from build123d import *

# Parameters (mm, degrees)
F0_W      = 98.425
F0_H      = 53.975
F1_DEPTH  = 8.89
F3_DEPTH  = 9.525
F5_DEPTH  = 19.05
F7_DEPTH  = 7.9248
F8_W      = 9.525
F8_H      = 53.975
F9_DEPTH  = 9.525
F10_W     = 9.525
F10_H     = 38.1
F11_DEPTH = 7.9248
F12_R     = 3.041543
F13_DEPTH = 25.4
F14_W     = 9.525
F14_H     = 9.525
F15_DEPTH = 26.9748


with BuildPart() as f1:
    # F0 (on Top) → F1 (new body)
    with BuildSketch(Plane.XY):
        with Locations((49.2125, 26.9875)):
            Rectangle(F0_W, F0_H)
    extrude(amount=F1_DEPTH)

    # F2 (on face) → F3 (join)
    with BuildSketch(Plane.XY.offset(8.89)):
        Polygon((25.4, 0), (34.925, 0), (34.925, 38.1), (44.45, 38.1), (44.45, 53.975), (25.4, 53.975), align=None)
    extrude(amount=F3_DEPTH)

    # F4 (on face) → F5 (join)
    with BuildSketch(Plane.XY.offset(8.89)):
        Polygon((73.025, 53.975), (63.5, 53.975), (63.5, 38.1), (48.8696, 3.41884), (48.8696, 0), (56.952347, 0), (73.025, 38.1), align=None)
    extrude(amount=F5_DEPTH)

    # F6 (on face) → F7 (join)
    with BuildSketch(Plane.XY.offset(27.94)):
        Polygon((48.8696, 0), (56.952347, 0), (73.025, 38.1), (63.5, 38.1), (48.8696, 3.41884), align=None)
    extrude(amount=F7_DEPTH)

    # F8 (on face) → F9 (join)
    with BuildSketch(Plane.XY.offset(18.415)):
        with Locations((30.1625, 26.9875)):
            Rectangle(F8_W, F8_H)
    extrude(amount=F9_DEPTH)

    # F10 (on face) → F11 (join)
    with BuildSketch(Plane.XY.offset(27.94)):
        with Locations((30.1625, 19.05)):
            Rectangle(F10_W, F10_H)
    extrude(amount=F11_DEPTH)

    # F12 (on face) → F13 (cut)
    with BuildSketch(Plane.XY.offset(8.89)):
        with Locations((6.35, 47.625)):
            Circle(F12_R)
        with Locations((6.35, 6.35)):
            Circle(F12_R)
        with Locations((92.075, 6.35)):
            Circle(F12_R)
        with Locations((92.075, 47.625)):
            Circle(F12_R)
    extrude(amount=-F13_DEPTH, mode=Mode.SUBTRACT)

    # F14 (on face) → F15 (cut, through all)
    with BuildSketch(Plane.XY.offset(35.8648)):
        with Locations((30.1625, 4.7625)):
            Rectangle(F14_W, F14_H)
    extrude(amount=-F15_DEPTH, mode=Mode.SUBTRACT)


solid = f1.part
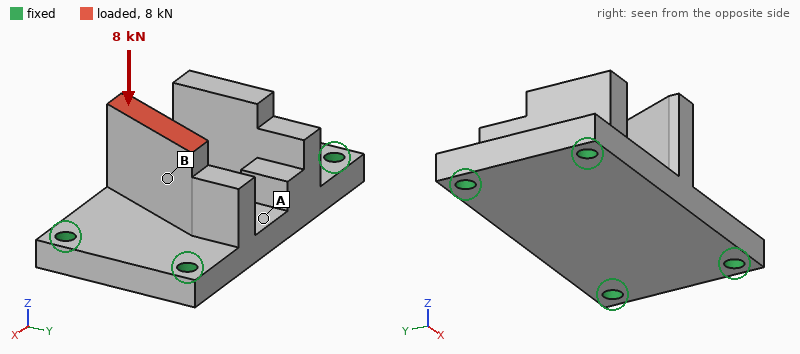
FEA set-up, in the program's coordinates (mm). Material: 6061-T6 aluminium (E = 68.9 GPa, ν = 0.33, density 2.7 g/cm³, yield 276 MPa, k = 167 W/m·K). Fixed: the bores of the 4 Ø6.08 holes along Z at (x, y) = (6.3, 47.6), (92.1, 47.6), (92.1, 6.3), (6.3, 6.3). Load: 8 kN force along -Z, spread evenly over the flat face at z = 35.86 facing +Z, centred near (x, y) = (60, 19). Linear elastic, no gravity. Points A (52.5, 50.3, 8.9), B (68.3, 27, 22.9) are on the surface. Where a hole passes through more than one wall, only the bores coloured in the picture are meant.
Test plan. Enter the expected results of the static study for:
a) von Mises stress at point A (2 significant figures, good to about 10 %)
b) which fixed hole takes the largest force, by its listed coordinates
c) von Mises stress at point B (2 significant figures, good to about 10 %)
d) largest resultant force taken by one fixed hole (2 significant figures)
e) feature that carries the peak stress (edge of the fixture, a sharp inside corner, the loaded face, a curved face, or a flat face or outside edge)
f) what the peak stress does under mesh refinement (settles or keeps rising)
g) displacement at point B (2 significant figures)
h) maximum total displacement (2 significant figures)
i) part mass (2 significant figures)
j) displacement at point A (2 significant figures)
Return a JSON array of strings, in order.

["58 MPa", "(92.1, 6.3)", "21 MPa", "3.4 kN", "edge of the fixture", "keeps rising", "0.10 mm", "0.20 mm", "190 g", "0.076 mm"]
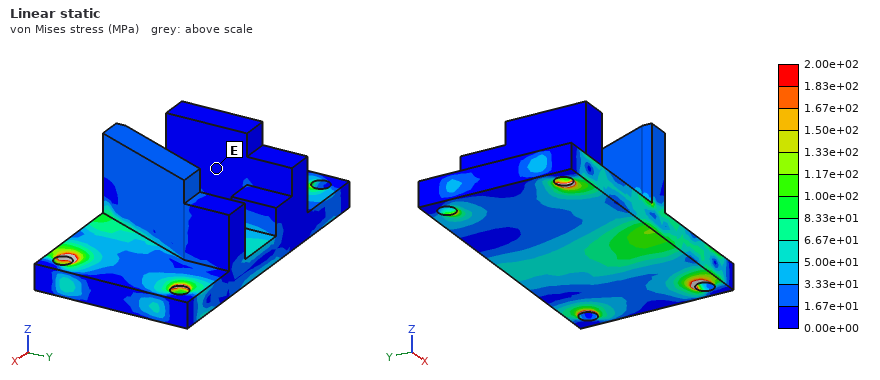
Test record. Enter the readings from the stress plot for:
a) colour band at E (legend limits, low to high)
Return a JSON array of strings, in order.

["0.00e+00 to 1.67e+01 MPa"]
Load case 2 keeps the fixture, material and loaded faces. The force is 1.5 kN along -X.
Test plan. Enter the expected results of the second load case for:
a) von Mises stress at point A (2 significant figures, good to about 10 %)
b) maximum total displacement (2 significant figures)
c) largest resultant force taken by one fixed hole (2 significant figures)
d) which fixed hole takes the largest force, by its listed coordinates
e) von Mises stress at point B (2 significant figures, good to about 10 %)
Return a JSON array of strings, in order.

["16 MPa", "0.10 mm", "640 N", "(92.1, 6.3)", "33 MPa"]
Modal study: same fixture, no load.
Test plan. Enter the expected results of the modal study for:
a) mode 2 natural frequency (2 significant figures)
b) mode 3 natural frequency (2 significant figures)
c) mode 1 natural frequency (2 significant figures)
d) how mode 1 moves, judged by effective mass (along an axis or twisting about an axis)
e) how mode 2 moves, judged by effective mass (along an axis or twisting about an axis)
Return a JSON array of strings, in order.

["5400 Hz", "7400 Hz", "3900 Hz", "along Z", "along Y"]
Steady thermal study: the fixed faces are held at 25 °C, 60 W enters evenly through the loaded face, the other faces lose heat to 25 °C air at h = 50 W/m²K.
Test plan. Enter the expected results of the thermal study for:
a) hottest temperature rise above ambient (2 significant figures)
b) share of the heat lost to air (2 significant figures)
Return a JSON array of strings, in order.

["39 K", "14 %"]
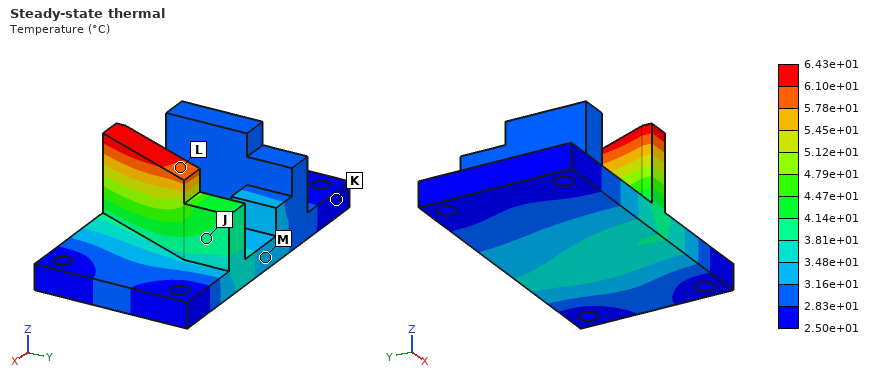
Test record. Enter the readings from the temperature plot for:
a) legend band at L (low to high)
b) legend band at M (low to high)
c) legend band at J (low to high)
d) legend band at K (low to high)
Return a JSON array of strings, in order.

["5.78e+01 to 6.10e+01 °C", "3.16e+01 to 3.48e+01 °C", "3.81e+01 to 4.14e+01 °C", "2.50e+01 to 2.83e+01 °C"]
